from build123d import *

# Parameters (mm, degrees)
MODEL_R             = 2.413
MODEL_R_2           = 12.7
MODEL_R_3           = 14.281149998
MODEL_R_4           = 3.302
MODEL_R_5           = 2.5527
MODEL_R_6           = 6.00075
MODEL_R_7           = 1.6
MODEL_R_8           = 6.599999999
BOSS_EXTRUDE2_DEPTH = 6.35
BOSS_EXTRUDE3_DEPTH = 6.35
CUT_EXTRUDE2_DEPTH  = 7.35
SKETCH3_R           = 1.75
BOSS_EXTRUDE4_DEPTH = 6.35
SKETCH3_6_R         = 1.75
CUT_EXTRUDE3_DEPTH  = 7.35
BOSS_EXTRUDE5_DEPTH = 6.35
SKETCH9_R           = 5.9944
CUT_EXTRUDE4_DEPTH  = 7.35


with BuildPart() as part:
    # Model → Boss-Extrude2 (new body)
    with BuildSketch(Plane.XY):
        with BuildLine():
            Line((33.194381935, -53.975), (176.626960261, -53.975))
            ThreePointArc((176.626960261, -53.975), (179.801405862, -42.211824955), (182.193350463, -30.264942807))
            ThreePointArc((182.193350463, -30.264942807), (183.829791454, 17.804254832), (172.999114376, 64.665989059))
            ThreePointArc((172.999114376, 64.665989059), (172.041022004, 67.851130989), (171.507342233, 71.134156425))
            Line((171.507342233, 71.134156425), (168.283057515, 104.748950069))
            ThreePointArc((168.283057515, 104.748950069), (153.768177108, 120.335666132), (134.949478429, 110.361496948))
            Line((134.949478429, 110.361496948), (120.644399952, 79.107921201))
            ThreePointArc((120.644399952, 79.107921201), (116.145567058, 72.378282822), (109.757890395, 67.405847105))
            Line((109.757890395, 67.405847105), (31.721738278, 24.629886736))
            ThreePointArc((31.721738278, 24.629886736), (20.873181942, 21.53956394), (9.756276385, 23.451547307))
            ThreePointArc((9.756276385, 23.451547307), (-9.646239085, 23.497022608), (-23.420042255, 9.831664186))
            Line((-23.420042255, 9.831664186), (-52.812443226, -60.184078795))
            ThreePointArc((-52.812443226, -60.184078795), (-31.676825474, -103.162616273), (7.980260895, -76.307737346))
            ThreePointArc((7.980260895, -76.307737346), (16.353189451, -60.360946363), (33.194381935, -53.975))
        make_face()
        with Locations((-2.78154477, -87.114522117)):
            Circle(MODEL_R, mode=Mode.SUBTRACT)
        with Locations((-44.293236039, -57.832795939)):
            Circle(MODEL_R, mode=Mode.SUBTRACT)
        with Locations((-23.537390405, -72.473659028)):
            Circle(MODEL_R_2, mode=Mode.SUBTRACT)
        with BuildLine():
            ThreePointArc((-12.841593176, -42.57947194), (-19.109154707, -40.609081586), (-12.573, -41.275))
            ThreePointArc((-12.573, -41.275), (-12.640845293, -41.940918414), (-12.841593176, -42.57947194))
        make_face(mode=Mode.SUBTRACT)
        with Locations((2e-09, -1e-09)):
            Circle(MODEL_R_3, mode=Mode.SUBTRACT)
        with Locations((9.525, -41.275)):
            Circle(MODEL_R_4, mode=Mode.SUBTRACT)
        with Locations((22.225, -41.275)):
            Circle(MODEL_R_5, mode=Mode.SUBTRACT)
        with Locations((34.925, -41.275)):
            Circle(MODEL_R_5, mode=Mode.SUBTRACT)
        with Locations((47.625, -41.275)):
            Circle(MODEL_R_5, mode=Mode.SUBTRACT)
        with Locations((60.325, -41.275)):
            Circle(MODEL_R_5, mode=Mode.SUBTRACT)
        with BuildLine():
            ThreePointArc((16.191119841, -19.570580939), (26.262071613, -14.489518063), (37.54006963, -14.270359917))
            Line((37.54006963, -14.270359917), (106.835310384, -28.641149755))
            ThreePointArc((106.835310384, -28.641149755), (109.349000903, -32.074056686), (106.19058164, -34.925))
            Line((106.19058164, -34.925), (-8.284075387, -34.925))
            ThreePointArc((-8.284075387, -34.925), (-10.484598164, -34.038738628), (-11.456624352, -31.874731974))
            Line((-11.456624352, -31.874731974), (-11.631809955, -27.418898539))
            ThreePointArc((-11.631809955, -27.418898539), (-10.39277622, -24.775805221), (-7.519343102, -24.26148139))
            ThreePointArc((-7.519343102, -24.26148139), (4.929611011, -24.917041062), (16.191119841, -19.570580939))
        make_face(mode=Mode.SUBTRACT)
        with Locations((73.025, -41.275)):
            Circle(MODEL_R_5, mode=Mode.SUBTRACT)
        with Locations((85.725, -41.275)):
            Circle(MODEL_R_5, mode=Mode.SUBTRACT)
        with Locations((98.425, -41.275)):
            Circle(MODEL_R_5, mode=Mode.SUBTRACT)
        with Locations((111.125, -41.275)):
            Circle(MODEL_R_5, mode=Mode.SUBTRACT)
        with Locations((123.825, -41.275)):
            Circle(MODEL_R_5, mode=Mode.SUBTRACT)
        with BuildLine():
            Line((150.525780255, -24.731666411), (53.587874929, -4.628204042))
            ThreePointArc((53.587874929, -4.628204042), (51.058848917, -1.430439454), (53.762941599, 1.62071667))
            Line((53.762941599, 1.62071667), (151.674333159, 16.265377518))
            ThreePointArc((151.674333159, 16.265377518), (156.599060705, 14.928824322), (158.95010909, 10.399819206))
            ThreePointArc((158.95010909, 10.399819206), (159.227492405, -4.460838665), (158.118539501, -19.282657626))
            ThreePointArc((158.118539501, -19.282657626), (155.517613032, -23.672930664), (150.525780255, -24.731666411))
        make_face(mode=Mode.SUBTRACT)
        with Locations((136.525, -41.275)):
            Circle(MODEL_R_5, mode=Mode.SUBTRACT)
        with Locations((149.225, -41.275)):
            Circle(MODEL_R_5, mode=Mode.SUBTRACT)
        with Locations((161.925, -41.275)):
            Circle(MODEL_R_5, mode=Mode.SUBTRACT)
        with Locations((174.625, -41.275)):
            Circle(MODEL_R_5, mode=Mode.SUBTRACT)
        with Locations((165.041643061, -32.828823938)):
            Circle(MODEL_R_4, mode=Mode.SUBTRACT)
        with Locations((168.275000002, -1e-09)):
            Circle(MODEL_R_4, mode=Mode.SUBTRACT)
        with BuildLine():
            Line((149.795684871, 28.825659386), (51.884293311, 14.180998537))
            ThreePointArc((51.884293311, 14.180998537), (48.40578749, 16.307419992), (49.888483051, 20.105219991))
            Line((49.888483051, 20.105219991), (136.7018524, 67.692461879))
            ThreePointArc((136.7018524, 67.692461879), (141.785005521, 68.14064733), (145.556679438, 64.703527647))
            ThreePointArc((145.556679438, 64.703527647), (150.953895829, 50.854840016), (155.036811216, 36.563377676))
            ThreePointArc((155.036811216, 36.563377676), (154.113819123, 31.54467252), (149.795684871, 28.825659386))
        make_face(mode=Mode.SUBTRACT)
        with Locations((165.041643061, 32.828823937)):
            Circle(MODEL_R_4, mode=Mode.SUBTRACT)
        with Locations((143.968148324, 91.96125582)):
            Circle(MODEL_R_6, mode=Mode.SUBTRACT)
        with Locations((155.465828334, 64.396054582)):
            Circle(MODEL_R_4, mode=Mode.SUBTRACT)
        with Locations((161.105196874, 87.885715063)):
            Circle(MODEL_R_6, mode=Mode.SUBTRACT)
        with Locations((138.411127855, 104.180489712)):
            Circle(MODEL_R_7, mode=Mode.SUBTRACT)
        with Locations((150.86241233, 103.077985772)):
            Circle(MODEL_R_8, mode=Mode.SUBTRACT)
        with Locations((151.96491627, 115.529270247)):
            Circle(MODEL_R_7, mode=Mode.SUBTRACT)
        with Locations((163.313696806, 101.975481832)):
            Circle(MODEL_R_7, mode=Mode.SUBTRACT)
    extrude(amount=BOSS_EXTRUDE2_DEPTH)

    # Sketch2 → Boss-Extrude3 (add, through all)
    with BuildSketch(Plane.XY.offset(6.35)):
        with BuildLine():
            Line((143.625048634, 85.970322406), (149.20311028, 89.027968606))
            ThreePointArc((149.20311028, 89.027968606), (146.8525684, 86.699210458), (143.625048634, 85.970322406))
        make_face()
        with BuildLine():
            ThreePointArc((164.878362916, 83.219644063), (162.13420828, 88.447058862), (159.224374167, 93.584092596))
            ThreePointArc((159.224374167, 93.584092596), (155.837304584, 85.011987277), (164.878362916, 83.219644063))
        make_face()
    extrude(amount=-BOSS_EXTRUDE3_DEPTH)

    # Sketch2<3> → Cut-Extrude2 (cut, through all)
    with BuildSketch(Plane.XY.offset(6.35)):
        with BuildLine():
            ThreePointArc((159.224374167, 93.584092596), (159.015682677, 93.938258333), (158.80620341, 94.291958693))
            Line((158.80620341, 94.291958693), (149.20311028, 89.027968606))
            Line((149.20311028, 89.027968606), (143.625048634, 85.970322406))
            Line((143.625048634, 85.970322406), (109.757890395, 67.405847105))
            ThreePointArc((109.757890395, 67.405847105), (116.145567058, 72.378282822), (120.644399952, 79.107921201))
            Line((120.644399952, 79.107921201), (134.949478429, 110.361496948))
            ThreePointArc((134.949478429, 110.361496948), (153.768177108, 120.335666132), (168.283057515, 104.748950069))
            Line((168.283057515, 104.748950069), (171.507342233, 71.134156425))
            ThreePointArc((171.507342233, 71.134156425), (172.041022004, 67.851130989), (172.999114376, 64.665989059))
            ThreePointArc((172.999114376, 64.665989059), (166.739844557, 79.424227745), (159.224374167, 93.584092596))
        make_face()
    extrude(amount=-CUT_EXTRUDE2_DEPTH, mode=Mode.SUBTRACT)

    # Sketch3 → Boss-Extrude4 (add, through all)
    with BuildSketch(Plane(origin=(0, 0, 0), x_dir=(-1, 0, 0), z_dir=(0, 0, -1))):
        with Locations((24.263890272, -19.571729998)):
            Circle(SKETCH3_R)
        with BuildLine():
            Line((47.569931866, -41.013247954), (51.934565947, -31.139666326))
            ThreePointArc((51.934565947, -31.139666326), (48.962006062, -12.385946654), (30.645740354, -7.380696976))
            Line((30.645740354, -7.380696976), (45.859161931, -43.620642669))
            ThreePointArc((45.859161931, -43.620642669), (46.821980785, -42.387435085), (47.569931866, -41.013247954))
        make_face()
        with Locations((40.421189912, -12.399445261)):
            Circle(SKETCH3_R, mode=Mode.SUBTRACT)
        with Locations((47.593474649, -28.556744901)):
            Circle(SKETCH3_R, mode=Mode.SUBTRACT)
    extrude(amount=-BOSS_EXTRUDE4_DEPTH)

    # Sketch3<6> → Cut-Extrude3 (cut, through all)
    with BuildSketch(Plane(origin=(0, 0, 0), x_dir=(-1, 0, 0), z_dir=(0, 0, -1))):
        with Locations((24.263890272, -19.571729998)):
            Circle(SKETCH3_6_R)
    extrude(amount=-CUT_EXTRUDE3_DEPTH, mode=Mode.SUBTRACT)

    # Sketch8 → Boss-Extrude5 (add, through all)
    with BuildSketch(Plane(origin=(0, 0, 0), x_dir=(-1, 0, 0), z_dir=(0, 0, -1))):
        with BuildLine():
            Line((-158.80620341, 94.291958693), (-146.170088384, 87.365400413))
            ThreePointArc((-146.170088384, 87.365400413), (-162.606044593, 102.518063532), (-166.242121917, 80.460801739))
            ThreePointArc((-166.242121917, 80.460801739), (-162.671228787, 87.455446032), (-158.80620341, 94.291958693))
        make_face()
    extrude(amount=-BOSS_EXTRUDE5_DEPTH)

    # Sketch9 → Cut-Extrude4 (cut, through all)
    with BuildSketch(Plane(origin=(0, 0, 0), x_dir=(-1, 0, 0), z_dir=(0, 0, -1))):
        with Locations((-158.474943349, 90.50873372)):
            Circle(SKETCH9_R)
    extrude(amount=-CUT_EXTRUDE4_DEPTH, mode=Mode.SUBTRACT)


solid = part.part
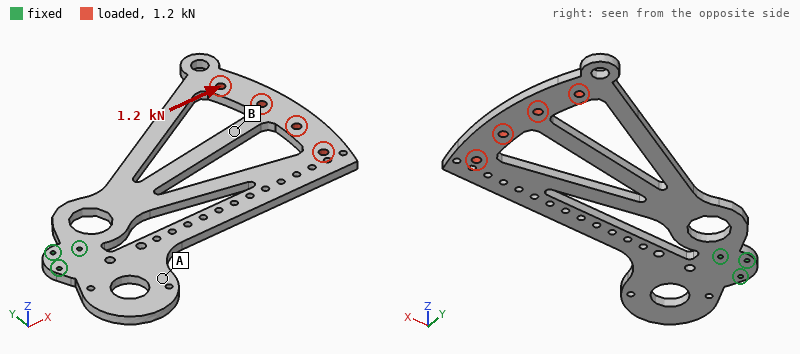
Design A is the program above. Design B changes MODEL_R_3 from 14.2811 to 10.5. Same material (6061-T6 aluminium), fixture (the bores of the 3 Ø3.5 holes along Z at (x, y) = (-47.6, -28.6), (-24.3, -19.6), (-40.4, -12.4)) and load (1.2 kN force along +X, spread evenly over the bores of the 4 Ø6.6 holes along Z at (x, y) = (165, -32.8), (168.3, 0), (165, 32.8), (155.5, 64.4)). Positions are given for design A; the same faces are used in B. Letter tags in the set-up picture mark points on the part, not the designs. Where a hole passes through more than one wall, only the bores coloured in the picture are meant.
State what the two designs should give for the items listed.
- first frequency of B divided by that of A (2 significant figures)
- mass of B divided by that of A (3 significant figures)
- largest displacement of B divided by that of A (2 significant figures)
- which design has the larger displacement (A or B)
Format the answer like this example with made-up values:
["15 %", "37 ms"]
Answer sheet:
["1.1", "1.02", "0.81", "A"]
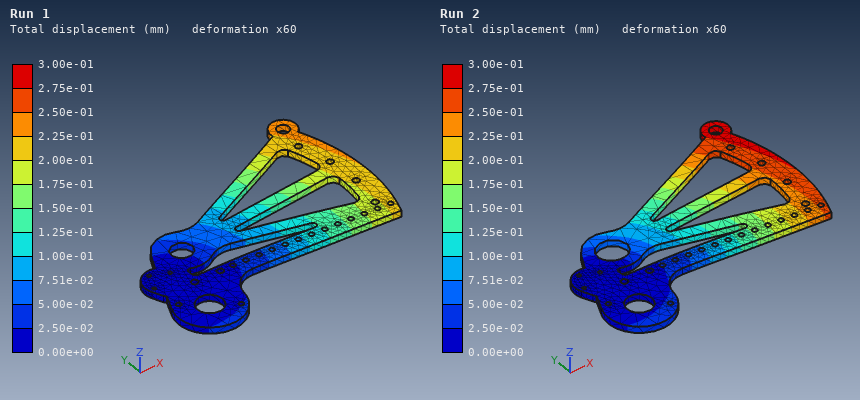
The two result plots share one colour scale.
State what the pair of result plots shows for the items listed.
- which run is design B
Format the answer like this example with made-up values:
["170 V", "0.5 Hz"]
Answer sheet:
["Run 1"]
